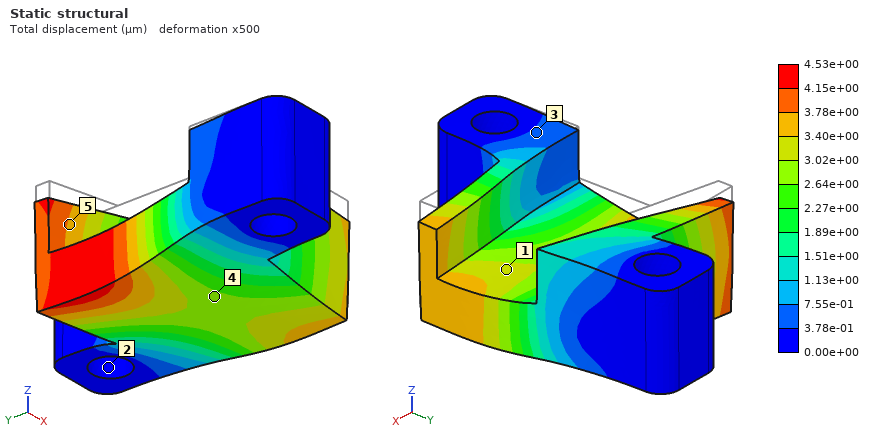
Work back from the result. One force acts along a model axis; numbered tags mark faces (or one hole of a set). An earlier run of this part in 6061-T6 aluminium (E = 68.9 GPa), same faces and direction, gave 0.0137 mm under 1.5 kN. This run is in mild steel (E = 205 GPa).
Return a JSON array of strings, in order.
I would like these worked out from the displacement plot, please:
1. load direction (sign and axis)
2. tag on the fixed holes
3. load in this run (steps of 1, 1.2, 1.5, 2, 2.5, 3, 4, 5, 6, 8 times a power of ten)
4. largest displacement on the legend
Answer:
["-Z", "2", "1.5 kN", "4.53e+00 µm"]
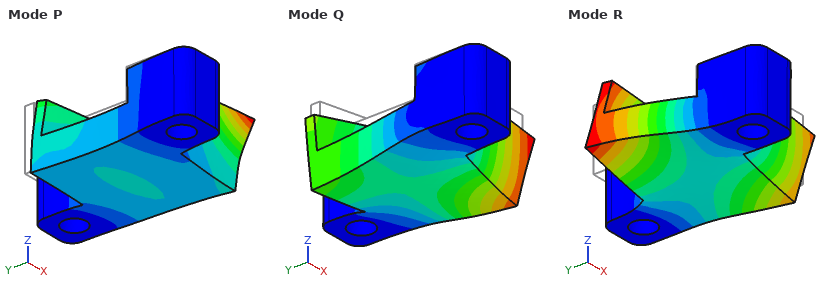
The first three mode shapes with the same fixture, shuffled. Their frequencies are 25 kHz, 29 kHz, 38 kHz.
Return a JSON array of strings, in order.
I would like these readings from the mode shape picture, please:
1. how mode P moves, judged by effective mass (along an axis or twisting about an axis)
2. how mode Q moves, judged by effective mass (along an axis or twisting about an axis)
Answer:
["along X", "along Z"]
